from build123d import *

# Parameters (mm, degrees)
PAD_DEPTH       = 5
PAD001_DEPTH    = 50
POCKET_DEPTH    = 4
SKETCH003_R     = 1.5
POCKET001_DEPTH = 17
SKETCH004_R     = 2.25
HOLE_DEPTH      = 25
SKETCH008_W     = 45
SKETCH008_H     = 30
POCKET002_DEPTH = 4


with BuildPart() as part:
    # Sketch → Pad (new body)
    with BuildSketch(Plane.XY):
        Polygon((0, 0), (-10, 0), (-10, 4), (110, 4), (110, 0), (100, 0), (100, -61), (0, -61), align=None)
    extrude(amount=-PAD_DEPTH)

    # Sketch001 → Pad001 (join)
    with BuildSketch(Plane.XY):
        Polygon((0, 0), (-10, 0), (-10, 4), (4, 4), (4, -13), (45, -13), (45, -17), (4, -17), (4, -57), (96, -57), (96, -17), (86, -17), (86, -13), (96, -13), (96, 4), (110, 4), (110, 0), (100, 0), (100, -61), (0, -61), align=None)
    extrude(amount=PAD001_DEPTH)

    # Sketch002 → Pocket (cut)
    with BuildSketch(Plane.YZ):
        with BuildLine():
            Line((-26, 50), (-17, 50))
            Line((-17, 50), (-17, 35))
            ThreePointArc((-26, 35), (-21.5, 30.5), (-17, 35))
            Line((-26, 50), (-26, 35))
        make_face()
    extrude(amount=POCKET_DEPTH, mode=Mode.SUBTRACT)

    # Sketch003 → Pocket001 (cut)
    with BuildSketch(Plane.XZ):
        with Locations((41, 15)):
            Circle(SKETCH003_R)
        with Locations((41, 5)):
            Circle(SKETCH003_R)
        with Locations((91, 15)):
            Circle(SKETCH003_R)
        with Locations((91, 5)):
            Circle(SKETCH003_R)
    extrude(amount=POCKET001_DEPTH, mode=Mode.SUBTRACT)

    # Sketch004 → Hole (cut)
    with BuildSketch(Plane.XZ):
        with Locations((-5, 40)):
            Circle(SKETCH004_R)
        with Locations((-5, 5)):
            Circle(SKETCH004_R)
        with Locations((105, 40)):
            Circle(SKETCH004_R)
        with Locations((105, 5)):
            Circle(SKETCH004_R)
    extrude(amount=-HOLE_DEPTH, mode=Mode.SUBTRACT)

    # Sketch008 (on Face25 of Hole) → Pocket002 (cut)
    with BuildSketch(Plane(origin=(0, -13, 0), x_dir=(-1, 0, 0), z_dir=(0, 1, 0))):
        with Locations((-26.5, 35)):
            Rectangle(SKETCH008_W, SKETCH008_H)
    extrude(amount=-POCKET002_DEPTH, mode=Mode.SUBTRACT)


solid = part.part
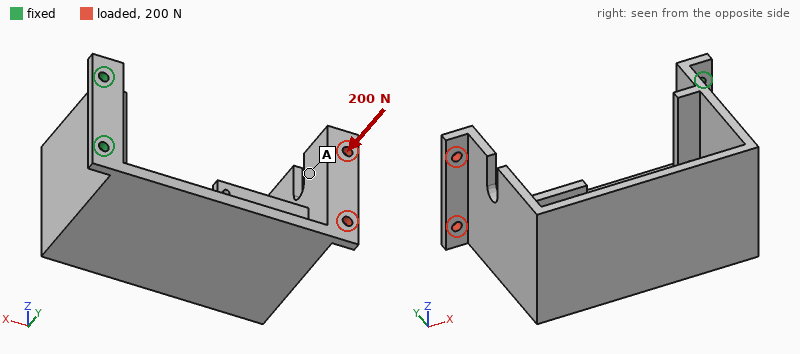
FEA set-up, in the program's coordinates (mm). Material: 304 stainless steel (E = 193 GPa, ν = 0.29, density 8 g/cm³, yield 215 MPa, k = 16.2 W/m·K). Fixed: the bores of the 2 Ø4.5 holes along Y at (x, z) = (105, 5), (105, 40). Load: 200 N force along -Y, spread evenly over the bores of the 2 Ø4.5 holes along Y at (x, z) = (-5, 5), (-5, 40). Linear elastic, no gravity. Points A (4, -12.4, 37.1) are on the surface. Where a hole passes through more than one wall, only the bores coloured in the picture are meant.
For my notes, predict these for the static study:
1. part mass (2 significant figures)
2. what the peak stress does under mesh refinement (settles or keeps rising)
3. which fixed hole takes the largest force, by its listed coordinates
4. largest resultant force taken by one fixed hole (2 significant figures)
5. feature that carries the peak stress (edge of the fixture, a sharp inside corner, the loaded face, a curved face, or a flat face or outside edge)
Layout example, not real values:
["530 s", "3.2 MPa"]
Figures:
["680 g", "keeps rising", "(105, 5)", "230 N", "edge of the fixture"]
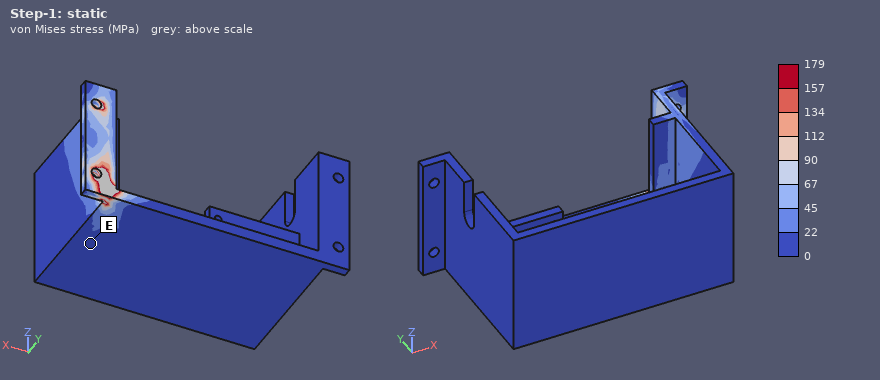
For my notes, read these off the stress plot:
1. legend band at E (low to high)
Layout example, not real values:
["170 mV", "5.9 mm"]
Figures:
["0 to 22 MPa"]
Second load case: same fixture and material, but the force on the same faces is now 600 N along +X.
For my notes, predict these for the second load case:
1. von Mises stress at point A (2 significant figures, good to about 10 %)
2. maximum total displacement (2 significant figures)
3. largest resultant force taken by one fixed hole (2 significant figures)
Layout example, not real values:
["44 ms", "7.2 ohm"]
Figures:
["19 MPa", "0.53 mm", "310 N"]
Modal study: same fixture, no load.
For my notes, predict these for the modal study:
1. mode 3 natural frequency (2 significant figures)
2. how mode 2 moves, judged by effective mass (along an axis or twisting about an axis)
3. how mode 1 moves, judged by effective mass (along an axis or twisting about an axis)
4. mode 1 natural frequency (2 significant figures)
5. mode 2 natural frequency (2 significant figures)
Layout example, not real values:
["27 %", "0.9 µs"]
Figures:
["720 Hz", "along Z", "along Y", "150 Hz", "250 Hz"]
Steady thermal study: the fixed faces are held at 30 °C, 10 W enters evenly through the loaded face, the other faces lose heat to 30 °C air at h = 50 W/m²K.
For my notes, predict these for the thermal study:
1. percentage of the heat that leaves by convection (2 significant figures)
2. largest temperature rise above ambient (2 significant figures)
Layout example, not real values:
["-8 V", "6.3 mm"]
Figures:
["100 %", "71 K"]
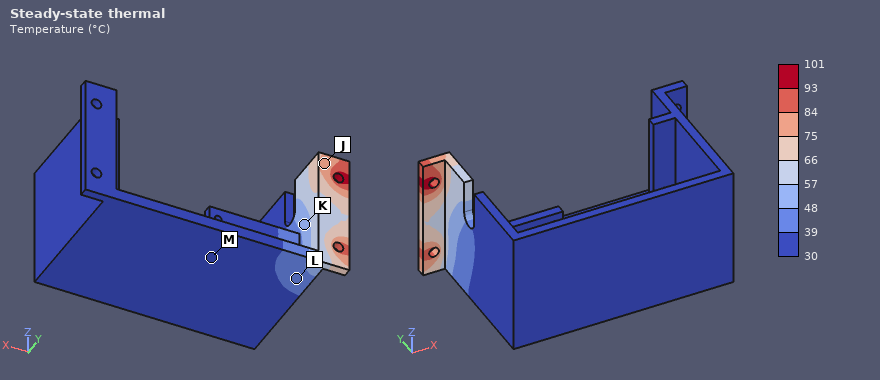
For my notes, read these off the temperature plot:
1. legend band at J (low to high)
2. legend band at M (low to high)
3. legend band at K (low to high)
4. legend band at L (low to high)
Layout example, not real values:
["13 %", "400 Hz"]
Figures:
["75 to 84 °C", "30 to 39 °C", "48 to 57 °C", "39 to 48 °C"]
